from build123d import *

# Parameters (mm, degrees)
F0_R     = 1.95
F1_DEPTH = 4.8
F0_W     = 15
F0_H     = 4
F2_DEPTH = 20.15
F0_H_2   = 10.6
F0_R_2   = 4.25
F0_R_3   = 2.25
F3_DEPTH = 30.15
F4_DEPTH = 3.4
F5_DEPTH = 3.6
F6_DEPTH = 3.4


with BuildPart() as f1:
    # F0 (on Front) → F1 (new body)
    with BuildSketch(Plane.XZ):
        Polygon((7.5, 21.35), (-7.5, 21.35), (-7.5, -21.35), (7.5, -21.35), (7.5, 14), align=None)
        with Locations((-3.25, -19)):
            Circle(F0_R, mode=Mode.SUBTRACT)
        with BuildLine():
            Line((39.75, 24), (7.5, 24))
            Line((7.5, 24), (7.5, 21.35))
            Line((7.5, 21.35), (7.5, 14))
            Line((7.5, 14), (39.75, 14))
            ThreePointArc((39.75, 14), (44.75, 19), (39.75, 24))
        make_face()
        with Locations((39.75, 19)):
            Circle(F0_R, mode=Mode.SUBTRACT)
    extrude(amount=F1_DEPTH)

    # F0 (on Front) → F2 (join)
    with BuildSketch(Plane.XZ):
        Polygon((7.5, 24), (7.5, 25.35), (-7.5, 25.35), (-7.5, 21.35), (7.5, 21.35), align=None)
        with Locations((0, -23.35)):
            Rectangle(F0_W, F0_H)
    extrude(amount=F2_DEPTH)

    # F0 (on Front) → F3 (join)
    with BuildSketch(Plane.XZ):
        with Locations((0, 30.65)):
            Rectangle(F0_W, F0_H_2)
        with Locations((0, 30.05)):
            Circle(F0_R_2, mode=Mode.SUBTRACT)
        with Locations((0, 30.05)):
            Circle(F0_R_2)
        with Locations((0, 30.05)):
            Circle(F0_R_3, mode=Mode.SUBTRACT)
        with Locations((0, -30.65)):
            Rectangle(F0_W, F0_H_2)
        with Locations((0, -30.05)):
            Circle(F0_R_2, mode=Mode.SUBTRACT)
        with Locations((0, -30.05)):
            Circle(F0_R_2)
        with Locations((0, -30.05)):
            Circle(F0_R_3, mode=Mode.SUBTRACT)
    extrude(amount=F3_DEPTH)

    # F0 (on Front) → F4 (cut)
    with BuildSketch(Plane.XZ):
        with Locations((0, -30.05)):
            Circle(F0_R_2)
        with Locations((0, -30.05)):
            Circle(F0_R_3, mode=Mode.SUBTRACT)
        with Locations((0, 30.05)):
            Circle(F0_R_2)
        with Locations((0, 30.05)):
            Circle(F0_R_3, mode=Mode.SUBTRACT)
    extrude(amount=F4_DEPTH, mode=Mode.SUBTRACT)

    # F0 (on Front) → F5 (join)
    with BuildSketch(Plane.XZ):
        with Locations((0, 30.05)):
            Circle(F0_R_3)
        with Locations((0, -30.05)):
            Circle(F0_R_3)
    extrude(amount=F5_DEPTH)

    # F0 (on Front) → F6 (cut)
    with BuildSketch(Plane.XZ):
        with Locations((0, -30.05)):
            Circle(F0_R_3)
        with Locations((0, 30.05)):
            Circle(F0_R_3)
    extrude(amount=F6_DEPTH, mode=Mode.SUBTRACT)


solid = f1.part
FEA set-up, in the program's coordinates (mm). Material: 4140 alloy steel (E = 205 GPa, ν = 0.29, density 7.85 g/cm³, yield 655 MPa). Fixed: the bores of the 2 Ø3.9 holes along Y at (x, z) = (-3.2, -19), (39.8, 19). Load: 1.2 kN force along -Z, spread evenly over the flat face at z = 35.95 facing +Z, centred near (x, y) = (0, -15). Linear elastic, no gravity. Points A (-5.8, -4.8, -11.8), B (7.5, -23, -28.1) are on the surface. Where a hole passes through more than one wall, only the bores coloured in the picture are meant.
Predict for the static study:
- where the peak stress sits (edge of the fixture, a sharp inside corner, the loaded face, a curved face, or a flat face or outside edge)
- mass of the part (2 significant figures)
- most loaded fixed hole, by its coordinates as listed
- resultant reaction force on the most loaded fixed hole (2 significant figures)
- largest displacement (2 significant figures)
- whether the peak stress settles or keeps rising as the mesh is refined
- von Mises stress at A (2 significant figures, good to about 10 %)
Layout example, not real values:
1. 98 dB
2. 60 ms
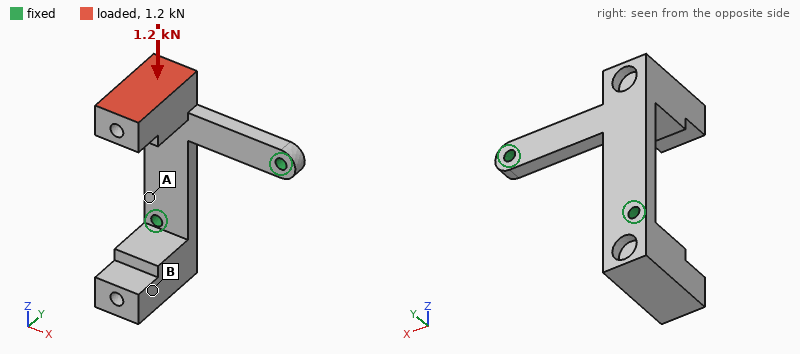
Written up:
1. edge of the fixture
2. 120 g
3. (-3.2, -19)
4. 1.2 kN
5. 0.43 mm
6. keeps rising
7. 98 MPa
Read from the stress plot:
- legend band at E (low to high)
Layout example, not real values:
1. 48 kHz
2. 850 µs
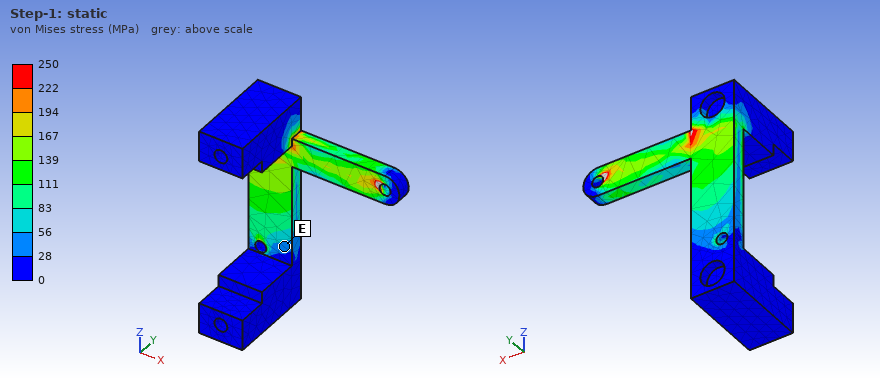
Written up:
1. 28 to 56 MPa
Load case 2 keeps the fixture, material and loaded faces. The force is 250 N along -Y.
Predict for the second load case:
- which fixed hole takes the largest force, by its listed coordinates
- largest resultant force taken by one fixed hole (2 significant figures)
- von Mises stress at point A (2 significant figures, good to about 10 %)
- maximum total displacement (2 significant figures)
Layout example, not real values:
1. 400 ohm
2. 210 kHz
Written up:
1. (39.8, 19)
2. 180 N
3. 83 MPa
4. 0.24 mm
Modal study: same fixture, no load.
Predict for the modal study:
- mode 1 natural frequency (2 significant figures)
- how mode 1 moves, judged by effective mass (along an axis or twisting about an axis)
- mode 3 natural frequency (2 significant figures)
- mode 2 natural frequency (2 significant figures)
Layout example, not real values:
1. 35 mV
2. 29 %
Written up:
1. 970 Hz
2. along Y
3. 3300 Hz
4. 2600 Hz
